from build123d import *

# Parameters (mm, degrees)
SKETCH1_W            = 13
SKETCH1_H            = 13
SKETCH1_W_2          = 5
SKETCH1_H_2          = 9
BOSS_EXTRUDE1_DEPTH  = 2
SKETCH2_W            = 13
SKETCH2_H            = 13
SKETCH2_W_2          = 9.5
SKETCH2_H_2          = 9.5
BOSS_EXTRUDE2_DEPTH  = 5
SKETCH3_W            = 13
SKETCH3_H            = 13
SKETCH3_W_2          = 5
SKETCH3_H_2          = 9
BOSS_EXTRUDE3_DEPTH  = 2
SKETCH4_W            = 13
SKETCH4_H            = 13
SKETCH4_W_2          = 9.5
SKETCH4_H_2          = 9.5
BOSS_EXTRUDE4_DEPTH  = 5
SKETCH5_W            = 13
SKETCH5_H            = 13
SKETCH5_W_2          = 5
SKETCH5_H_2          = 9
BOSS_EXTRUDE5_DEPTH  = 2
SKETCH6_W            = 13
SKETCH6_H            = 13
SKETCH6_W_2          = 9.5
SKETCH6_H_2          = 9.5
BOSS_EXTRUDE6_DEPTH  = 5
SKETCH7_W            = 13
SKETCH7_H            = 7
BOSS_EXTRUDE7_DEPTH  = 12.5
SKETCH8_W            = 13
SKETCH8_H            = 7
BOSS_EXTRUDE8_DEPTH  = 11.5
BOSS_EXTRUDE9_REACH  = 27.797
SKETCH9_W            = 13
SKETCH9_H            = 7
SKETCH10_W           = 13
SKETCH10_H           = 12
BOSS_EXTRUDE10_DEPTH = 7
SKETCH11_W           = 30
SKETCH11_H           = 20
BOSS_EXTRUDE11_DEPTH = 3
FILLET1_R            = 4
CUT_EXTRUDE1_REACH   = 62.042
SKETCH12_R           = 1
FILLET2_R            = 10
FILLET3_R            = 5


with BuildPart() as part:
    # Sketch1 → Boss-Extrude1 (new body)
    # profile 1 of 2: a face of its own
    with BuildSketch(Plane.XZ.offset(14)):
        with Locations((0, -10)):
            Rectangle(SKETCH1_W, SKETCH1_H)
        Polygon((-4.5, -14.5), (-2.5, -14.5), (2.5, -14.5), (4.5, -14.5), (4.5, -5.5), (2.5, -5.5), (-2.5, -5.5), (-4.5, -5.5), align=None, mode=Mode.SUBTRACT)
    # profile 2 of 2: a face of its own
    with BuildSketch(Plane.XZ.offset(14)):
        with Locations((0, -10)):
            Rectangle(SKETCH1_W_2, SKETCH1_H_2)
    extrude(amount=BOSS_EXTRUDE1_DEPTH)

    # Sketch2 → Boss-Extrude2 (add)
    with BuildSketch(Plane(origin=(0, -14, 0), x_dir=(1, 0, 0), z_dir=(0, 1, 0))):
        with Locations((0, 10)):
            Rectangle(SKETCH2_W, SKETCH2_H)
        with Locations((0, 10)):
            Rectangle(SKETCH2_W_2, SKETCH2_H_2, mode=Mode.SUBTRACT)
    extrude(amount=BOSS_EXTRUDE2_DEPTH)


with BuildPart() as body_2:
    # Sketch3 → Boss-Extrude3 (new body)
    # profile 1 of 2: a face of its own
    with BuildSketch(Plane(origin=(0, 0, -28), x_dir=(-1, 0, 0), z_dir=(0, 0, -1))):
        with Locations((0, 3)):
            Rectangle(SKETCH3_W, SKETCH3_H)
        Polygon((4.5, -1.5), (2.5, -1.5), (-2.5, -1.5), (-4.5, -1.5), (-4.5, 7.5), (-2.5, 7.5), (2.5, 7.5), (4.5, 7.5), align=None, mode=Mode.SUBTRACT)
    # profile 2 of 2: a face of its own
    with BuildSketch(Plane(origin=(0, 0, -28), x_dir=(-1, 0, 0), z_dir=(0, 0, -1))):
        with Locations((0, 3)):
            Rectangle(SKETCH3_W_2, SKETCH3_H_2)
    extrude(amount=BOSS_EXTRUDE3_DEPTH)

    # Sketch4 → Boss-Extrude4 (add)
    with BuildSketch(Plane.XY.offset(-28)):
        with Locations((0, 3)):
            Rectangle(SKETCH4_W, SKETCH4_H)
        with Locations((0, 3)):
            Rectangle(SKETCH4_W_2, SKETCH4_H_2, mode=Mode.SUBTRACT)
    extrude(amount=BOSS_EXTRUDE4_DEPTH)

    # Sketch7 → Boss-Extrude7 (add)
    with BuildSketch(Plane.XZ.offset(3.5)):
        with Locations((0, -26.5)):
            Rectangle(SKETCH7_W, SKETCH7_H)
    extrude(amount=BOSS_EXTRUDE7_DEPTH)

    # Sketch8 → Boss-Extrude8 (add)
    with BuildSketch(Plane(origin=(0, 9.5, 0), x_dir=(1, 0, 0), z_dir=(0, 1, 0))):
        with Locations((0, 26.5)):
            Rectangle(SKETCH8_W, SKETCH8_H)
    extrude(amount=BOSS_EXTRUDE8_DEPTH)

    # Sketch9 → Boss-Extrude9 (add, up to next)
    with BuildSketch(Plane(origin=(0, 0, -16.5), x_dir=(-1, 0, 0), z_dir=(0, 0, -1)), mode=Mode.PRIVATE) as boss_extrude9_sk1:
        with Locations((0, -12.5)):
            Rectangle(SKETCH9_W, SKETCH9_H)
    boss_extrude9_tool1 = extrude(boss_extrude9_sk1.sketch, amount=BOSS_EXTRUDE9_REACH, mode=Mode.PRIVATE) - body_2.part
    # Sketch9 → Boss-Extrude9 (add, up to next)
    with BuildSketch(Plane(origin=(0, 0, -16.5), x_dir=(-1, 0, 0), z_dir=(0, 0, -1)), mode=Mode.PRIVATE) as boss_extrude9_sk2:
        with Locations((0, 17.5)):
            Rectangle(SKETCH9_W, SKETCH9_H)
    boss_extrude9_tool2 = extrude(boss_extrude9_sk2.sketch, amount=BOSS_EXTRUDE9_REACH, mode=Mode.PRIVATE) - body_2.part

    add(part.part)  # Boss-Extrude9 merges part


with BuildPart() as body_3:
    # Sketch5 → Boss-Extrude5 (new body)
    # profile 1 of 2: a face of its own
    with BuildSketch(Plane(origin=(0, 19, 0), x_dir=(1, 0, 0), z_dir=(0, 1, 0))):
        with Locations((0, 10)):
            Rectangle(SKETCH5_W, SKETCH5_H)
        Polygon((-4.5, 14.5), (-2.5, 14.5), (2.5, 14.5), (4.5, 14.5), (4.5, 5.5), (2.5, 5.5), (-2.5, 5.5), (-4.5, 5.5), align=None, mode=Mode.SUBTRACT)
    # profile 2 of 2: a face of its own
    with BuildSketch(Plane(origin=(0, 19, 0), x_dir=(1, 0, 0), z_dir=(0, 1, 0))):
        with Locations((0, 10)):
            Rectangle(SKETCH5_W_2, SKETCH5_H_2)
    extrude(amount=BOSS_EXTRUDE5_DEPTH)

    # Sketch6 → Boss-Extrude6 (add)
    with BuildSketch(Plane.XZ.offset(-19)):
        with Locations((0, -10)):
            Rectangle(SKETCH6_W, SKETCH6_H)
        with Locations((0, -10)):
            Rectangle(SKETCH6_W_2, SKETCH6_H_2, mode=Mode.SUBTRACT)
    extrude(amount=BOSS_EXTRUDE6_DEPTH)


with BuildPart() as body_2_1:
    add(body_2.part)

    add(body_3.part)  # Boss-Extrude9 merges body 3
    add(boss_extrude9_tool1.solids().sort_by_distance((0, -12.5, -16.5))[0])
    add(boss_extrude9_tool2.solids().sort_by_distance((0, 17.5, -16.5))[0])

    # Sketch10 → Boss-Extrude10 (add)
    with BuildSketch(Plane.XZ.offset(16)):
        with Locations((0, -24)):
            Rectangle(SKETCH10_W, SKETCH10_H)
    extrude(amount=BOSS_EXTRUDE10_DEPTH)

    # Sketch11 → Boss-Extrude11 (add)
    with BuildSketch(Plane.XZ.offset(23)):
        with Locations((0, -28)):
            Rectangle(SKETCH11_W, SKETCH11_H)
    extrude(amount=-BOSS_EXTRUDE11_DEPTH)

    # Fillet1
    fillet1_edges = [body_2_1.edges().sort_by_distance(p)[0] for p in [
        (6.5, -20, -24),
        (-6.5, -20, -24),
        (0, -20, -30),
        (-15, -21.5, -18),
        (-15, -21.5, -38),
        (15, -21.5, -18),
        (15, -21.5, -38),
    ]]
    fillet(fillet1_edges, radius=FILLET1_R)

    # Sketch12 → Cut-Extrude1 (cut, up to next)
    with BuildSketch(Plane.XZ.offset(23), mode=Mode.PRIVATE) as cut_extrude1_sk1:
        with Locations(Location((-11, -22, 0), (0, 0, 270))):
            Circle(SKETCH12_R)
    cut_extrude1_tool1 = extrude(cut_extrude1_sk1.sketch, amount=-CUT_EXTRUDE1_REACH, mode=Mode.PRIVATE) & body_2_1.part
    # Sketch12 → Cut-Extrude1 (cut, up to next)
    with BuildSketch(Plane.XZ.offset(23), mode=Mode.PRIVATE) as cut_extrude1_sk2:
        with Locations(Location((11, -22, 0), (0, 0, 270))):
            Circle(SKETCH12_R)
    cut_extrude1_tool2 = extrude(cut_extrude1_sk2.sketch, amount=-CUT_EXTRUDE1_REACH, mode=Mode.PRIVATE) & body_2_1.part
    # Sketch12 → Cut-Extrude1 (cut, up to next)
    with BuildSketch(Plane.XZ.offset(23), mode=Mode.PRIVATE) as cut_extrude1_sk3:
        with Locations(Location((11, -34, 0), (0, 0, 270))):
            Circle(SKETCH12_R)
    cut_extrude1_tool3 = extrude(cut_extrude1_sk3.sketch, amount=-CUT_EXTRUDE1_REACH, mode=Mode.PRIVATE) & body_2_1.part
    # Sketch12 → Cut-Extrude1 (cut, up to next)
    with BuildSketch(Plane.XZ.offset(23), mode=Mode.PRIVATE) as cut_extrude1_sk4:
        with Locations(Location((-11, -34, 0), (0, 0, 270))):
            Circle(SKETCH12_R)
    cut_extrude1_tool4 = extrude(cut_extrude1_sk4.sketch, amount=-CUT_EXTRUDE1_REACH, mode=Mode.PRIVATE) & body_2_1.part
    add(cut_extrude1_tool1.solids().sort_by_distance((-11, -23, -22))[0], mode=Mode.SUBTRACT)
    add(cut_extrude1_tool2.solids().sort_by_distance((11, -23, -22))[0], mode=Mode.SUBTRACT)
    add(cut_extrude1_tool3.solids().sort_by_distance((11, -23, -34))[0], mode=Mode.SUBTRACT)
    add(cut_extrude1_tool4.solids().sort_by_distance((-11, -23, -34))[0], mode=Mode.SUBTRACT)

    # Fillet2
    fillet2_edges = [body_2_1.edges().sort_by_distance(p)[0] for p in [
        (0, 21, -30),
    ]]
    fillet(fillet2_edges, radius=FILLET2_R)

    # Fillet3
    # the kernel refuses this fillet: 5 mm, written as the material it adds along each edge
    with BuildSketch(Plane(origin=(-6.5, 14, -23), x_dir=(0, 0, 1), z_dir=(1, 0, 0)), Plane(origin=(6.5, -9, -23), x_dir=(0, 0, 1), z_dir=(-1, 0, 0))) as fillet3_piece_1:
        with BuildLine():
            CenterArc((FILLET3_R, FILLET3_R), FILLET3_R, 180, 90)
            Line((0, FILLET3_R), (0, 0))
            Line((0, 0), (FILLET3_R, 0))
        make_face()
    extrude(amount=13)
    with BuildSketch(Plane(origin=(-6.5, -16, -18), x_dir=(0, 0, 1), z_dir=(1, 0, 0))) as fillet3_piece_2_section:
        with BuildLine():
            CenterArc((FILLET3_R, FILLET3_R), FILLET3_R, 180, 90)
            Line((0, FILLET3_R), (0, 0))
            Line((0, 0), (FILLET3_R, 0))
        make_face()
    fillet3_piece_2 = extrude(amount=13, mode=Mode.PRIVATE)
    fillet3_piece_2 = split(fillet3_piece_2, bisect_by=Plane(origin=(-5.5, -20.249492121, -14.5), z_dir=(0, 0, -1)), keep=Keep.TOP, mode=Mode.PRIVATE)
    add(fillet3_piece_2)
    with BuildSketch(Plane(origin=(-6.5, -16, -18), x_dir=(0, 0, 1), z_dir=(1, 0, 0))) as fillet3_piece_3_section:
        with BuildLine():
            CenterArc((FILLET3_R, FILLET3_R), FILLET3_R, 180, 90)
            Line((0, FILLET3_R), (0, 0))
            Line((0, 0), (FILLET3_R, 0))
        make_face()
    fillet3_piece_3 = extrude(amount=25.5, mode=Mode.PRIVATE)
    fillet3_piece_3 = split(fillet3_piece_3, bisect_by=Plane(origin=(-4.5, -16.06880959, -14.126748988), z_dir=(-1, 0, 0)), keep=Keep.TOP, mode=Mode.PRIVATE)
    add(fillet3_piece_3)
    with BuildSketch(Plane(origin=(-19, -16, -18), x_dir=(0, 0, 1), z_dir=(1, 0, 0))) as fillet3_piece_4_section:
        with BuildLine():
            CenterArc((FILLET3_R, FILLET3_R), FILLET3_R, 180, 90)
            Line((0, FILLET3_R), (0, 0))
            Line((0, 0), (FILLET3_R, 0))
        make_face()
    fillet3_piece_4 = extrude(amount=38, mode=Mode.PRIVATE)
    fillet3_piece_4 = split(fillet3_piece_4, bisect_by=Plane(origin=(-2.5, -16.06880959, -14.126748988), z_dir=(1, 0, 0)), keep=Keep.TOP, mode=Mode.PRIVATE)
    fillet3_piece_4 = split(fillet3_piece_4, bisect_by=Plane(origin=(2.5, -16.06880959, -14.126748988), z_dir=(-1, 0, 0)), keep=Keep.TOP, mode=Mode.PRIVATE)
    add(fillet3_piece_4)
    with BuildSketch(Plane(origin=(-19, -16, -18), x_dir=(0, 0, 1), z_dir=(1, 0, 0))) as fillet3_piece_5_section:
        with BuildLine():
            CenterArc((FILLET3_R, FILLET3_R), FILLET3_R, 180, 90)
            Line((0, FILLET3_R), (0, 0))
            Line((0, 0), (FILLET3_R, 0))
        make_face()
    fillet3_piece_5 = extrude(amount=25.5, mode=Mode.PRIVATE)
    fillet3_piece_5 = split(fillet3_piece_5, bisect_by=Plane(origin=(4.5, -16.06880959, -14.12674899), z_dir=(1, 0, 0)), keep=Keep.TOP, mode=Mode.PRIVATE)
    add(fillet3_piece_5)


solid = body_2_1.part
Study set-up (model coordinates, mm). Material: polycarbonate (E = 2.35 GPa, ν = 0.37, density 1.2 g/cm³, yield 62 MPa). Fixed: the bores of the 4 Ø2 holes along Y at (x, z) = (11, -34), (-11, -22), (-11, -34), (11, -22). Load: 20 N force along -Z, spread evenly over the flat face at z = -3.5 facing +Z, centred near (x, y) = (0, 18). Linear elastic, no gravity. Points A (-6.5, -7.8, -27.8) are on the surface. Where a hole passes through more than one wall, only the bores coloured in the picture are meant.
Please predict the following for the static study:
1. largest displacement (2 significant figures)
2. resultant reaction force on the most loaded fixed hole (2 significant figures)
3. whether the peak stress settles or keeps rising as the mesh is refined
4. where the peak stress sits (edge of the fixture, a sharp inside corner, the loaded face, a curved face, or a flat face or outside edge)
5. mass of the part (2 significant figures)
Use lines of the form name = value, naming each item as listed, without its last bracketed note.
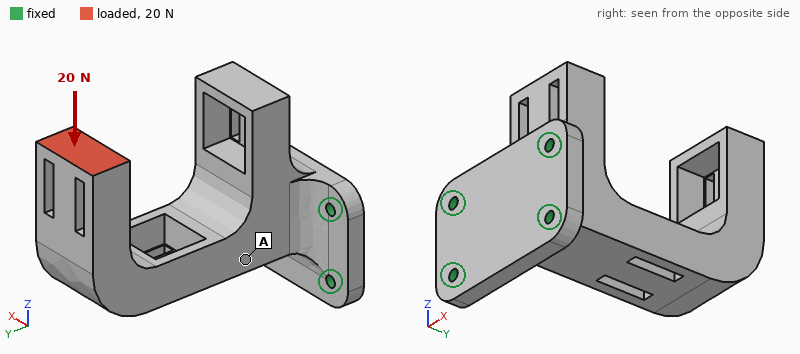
largest displacement = 0.68 mm
resultant reaction force on the most loaded fixed hole = 34 N
whether the peak stress settles or keeps rising as the mesh is refined = keeps rising
where the peak stress sits = edge of the fixture
mass of the part = 9.3 g
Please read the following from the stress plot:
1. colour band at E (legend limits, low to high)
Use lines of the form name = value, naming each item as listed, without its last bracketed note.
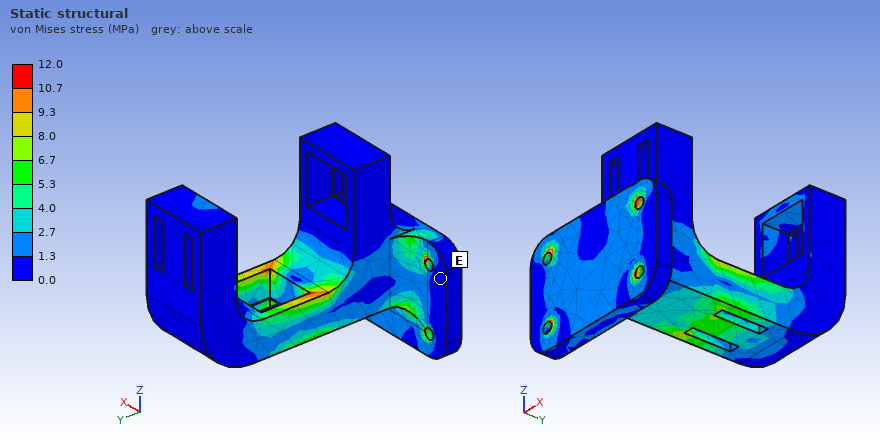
colour band at E = 0.0 to 1.3 MPa
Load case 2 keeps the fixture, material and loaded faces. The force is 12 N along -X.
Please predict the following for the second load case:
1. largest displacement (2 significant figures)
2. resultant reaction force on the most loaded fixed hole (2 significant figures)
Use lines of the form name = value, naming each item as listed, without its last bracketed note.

largest displacement = 0.66 mm
resultant reaction force on the most loaded fixed hole = 19 N
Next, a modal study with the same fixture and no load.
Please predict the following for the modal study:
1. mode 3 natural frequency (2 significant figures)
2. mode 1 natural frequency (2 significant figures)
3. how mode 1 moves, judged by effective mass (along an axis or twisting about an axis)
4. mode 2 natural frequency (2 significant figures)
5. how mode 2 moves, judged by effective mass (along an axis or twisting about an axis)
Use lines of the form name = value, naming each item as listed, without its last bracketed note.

mode 3 natural frequency = 1800 Hz
mode 1 natural frequency = 610 Hz
how mode 1 moves, judged by effective mass = along Z
mode 2 natural frequency = 760 Hz
how mode 2 moves, judged by effective mass = along X
